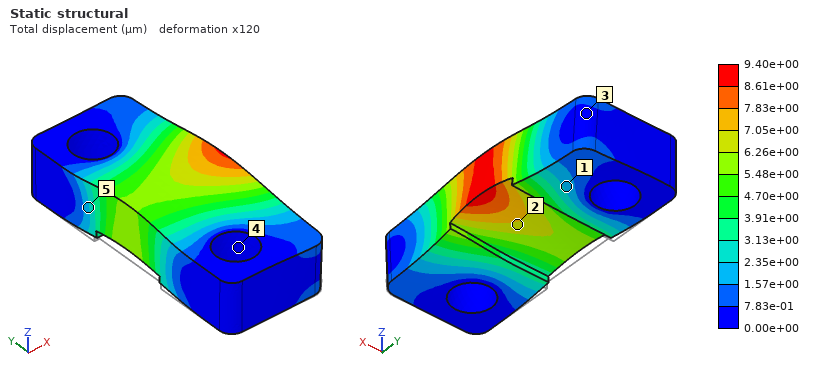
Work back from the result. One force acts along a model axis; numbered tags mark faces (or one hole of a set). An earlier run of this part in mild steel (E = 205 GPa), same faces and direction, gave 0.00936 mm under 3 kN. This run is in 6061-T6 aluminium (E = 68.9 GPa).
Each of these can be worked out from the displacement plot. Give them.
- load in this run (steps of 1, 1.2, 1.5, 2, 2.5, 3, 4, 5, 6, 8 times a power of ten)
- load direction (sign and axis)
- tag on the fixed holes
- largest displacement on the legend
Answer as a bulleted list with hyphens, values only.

- 1 kN
- +Z
- 4
- 9.40e+00 µm
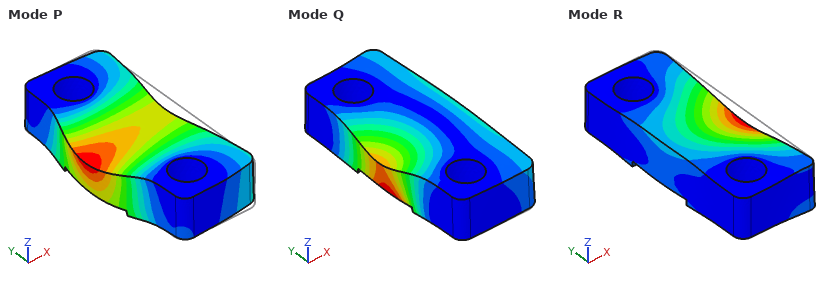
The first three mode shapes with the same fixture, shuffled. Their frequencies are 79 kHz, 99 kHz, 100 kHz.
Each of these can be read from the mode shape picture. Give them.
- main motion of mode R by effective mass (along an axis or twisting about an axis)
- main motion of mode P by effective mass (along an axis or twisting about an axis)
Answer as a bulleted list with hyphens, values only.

- along Z
- along X
